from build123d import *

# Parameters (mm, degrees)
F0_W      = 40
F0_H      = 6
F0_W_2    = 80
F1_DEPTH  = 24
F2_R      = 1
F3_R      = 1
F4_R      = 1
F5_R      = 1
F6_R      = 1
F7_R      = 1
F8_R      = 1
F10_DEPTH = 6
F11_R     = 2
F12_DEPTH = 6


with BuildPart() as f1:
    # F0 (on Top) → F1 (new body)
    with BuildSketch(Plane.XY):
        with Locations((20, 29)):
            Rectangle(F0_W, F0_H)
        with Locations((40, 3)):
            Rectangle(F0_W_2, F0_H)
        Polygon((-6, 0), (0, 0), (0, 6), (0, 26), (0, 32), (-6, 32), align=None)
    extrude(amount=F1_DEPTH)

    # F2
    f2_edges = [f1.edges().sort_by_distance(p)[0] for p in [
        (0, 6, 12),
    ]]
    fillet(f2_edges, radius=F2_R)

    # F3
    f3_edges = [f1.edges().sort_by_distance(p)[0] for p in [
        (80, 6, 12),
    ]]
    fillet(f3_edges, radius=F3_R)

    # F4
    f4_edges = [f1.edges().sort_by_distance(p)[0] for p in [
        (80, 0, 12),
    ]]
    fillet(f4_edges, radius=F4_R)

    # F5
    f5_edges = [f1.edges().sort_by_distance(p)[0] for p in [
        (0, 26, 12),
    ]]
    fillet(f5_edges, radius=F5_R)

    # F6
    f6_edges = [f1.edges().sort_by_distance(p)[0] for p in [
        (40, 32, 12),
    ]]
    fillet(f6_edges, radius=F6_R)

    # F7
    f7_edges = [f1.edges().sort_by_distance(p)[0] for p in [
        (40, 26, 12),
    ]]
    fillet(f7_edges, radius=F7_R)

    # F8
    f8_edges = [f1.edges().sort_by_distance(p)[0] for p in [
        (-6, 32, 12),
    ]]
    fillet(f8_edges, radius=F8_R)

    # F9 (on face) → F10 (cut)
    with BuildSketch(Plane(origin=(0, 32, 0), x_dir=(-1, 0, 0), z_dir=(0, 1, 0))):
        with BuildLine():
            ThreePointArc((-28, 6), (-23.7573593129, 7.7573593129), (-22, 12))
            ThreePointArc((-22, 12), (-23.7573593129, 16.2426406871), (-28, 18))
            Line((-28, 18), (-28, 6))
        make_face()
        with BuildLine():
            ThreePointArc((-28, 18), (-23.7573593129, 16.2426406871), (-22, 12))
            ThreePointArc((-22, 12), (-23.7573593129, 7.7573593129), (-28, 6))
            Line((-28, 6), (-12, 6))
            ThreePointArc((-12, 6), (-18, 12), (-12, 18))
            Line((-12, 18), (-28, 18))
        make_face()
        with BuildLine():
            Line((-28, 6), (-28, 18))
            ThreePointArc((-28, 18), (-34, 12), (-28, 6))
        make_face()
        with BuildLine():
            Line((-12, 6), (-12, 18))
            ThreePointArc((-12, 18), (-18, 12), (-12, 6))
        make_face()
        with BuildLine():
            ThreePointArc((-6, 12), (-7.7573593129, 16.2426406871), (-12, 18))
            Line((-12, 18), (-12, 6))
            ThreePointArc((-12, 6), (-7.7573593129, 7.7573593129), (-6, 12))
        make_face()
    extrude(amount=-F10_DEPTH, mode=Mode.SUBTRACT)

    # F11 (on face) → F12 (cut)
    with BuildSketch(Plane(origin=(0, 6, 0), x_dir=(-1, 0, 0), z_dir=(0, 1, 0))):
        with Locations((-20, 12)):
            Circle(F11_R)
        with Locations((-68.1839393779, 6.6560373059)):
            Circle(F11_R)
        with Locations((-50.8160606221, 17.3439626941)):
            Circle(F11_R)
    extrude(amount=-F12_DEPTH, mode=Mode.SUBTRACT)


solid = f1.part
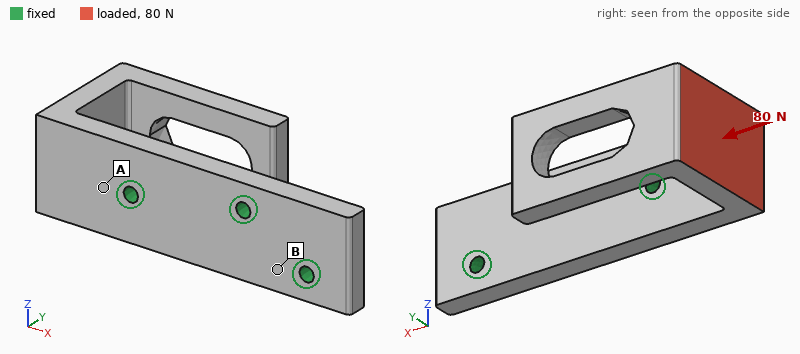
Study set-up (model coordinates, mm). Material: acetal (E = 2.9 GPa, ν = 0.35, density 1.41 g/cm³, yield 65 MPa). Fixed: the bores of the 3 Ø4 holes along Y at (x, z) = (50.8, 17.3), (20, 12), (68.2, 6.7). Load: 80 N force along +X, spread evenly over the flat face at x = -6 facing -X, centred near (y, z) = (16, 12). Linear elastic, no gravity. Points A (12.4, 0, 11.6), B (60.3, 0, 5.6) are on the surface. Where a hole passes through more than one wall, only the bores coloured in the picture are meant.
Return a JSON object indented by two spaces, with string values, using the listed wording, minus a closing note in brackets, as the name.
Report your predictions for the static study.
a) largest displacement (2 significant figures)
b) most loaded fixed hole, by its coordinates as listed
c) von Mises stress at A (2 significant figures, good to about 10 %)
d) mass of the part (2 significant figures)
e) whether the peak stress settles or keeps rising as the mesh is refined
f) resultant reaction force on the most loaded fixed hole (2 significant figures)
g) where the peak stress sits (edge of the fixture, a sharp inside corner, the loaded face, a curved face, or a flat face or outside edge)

{
  "largest displacement": "1.0 mm",
  "most loaded fixed hole, by its coordinates as listed": "(20, 12)",
  "von Mises stress at A": "6.0 MPa",
  "mass of the part": "28 g",
  "whether the peak stress settles or keeps rising as the mesh is refined": "keeps rising",
  "resultant reaction force on the most loaded fixed hole": "68 N",
  "where the peak stress sits": "edge of the fixture"
}
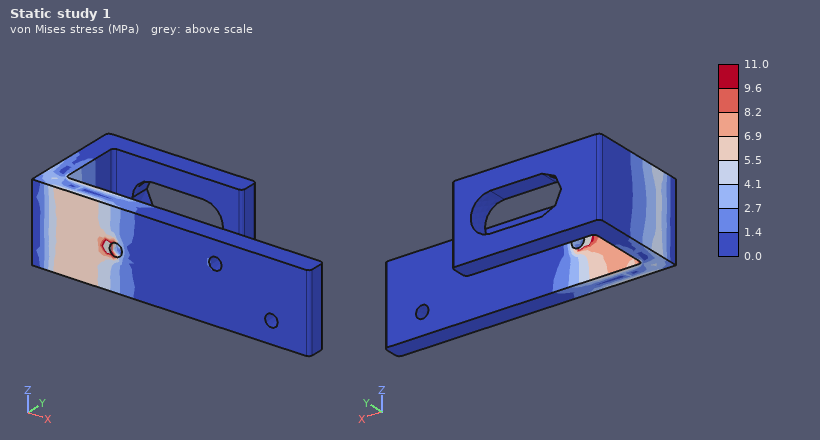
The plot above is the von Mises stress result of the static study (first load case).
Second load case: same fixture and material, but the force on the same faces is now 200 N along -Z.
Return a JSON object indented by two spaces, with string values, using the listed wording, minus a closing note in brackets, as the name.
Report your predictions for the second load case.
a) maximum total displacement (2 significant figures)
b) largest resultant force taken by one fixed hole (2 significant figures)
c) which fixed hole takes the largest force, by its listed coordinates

{
  "maximum total displacement": "1.1 mm",
  "largest resultant force taken by one fixed hole": "330 N",
  "which fixed hole takes the largest force, by its listed coordinates": "(20, 12)"
}
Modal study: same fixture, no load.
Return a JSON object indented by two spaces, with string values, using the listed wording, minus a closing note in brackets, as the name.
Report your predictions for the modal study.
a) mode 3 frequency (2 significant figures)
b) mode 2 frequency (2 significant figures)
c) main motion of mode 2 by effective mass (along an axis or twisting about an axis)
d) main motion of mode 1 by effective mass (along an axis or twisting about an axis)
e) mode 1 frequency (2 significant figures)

{
  "mode 3 frequency": "670 Hz",
  "mode 2 frequency": "440 Hz",
  "main motion of mode 2 by effective mass": "along Z",
  "main motion of mode 1 by effective mass": "along X",
  "mode 1 frequency": "330 Hz"
}
